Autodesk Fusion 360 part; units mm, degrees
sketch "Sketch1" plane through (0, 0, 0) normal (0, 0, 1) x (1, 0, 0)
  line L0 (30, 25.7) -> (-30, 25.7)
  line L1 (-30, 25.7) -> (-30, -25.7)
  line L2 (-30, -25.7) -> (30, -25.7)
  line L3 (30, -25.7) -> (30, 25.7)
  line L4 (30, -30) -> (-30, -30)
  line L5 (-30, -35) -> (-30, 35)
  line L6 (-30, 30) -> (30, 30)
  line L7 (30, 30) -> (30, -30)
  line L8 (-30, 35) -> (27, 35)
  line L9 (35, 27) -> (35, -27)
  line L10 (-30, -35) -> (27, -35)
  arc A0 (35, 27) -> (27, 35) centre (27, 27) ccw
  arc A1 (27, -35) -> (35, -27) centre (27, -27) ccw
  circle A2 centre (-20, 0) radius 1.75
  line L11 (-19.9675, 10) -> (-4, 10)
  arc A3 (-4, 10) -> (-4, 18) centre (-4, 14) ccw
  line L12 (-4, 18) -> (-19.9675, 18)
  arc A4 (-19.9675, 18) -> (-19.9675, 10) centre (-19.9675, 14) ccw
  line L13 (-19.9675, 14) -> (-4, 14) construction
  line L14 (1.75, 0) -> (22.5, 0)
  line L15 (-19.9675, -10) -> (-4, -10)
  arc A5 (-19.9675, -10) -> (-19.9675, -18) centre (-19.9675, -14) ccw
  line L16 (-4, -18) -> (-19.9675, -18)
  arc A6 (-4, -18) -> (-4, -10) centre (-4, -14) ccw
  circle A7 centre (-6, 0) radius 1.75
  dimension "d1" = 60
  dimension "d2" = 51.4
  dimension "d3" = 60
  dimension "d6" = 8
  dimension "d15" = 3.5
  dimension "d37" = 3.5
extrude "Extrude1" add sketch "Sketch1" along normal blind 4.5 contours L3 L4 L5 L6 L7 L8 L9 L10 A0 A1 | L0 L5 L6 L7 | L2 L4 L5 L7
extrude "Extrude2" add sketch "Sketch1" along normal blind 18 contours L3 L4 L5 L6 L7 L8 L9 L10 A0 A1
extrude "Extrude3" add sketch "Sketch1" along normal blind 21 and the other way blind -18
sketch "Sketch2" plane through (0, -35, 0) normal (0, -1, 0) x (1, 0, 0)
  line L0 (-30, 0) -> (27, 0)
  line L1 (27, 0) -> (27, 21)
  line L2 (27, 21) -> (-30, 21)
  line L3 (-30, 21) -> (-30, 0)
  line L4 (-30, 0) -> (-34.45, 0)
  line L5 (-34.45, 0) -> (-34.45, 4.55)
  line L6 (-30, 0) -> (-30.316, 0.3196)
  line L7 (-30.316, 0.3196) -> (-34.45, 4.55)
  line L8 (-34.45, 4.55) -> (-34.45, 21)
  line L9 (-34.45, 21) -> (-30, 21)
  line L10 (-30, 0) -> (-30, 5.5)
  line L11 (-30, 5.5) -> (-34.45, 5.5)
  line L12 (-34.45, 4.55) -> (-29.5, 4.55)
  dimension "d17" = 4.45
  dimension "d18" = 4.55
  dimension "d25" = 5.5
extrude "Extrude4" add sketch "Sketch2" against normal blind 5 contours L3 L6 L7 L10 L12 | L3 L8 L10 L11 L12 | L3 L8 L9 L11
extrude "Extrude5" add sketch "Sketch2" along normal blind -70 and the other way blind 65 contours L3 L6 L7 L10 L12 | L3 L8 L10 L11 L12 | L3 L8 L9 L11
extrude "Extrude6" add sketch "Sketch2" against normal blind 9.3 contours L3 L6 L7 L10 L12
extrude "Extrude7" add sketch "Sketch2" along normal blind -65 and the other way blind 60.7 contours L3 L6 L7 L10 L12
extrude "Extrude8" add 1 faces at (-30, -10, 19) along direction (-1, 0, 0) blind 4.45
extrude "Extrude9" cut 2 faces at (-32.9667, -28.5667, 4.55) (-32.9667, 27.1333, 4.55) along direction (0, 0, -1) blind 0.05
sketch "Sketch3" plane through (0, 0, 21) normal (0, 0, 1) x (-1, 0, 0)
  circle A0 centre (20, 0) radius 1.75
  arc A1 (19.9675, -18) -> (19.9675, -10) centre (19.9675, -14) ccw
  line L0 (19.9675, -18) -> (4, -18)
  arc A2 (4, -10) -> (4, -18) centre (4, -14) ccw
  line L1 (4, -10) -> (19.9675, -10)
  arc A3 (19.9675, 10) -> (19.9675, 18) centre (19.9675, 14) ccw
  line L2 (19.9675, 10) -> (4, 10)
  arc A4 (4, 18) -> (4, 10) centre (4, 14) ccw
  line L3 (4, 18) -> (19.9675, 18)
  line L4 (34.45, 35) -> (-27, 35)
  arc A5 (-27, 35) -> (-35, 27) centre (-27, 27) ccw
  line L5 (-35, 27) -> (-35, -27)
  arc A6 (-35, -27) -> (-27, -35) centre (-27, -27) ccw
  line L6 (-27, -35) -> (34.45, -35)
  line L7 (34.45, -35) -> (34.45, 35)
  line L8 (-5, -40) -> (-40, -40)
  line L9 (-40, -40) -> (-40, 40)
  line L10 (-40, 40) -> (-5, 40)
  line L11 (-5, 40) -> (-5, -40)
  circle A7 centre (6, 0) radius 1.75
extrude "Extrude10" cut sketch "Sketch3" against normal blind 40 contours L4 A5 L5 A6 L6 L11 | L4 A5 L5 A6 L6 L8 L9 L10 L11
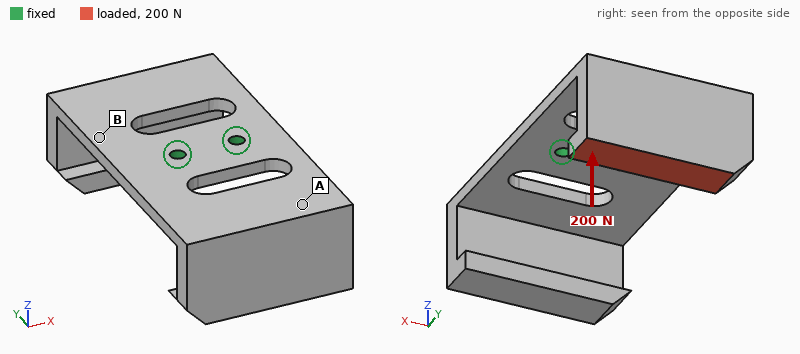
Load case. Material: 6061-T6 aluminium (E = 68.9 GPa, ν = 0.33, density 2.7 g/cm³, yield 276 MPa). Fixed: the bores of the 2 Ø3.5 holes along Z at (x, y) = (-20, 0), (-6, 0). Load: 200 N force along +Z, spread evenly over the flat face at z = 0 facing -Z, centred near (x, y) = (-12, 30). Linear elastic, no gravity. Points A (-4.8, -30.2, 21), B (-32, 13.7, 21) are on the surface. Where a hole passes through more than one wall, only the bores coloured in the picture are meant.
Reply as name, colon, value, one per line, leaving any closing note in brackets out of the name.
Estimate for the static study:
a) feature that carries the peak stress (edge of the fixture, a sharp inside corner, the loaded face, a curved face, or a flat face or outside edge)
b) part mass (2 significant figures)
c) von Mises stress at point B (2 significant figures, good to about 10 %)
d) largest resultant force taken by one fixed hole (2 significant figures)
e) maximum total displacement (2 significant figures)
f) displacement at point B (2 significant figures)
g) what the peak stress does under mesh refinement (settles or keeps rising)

feature that carries the peak stress: edge of the fixture
part mass: 42 g
von Mises stress at point B: 110 MPa
largest resultant force taken by one fixed hole: 100 N
maximum total displacement: 0.88 mm
displacement at point B: 0.14 mm
what the peak stress does under mesh refinement: keeps rising
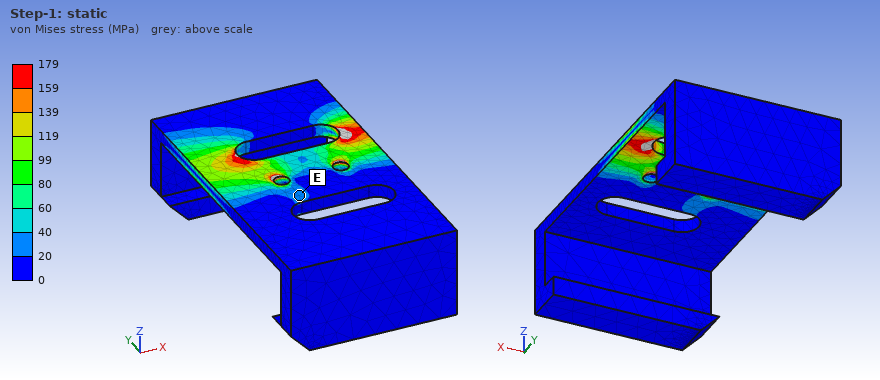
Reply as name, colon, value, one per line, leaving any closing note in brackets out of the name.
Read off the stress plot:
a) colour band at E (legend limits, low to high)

colour band at E: 20 to 40 MPa
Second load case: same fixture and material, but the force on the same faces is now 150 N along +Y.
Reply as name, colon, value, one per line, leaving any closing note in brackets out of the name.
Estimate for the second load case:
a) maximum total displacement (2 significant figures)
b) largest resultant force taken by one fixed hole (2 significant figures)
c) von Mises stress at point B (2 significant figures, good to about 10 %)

maximum total displacement: 0.73 mm
largest resultant force taken by one fixed hole: 78 N
von Mises stress at point B: 100 MPa
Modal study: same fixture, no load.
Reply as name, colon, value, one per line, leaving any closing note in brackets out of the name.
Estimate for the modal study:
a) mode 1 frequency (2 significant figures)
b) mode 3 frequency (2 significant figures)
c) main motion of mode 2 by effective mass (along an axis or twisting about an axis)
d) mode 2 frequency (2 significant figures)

mode 1 frequency: 620 Hz
mode 3 frequency: 1500 Hz
main motion of mode 2 by effective mass: along Z
mode 2 frequency: 670 Hz
